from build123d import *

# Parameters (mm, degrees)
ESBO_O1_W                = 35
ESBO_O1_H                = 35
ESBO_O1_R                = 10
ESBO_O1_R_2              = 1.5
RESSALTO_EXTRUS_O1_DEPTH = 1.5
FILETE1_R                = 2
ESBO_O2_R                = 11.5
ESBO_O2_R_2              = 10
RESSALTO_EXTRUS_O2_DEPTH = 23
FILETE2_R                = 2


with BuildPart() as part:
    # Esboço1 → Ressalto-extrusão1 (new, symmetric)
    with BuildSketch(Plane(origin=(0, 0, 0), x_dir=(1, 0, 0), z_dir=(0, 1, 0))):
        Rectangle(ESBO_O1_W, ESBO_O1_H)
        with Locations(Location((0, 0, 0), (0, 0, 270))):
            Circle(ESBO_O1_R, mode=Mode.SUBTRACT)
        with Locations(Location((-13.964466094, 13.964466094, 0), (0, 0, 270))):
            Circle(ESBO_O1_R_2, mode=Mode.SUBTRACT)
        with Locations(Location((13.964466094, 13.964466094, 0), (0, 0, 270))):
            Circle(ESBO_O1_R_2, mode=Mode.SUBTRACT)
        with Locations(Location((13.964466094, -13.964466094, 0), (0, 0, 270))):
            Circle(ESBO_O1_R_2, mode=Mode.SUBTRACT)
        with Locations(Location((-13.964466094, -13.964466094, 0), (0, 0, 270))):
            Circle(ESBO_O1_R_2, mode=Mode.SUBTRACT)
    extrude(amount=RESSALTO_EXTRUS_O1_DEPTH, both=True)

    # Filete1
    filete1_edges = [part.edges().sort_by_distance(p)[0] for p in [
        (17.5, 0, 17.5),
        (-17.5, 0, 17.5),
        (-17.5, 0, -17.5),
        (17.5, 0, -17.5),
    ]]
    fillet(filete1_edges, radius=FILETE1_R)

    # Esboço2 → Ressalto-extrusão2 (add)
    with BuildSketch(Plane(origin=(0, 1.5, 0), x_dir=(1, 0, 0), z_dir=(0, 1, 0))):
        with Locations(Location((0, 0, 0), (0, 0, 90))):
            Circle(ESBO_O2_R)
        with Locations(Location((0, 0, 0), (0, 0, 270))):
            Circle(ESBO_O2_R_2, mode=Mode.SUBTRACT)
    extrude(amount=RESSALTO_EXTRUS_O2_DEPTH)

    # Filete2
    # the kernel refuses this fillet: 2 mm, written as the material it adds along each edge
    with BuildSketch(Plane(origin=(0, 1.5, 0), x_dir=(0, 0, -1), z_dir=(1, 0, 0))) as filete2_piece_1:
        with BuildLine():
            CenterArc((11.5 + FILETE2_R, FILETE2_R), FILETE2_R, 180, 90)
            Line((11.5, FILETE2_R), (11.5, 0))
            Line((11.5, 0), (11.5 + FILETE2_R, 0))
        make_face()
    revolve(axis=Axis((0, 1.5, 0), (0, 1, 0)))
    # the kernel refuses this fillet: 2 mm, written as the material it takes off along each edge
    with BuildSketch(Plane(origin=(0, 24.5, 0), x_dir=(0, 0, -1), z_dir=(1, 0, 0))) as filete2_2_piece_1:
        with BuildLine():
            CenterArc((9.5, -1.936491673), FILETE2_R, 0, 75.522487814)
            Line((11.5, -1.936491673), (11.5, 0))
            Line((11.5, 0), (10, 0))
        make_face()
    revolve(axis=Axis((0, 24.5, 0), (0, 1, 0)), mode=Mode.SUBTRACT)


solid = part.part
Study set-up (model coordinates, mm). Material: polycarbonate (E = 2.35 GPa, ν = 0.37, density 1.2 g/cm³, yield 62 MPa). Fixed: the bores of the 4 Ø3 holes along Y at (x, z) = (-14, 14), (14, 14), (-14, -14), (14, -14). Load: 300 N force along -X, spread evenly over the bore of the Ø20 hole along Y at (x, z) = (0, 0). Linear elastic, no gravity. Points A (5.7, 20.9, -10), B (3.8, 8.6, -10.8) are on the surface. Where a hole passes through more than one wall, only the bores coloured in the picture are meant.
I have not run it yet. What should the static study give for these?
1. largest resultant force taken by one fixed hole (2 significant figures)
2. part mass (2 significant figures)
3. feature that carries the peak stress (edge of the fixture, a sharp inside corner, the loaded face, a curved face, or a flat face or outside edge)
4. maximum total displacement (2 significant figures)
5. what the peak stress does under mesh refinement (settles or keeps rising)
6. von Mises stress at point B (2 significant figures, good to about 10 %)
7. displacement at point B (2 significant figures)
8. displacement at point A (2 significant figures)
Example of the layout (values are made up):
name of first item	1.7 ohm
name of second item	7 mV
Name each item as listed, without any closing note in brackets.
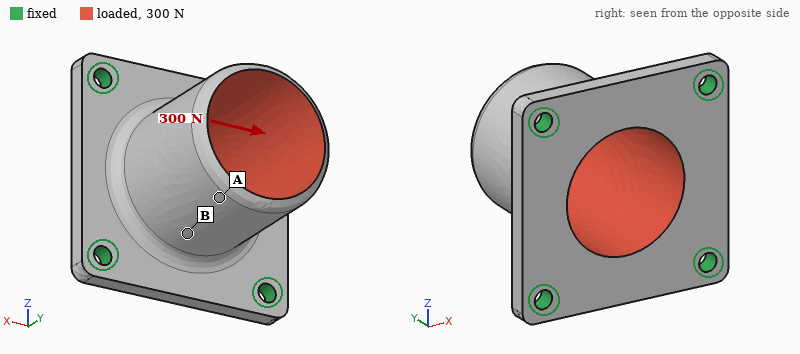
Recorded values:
largest resultant force taken by one fixed hole	110 N
part mass	6.0 g
feature that carries the peak stress	edge of the fixture
maximum total displacement	0.38 mm
what the peak stress does under mesh refinement	keeps rising
von Mises stress at point B	4.9 MPa
displacement at point B	0.13 mm
displacement at point A	0.31 mm
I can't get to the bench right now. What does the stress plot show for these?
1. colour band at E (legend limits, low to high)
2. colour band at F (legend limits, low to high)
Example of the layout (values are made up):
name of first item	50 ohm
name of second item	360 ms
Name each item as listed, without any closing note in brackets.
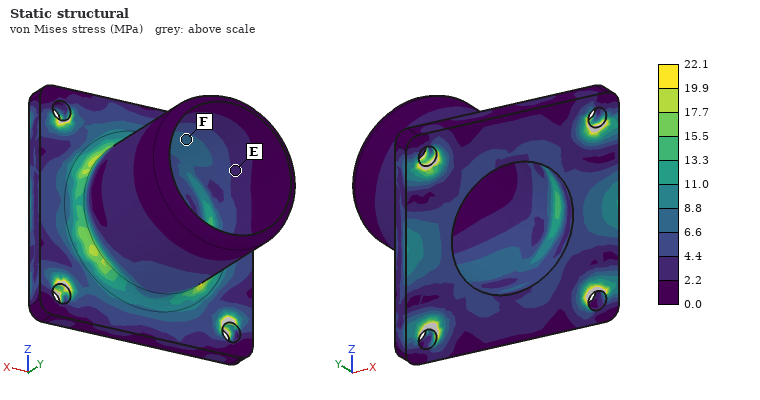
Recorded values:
colour band at E	2.2 to 4.4 MPa
colour band at F	6.6 to 8.8 MPa
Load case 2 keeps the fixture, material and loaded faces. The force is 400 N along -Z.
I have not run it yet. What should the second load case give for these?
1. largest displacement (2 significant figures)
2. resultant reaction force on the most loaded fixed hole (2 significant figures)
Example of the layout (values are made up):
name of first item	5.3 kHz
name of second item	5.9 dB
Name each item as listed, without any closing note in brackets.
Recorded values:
largest displacement	0.50 mm
resultant reaction force on the most loaded fixed hole	150 N
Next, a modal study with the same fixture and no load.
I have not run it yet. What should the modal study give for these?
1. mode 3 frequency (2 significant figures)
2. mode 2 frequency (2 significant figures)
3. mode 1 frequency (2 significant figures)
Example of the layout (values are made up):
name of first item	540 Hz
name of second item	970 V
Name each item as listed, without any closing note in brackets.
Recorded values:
mode 3 frequency	3000 Hz
mode 2 frequency	2800 Hz
mode 1 frequency	2800 Hz
